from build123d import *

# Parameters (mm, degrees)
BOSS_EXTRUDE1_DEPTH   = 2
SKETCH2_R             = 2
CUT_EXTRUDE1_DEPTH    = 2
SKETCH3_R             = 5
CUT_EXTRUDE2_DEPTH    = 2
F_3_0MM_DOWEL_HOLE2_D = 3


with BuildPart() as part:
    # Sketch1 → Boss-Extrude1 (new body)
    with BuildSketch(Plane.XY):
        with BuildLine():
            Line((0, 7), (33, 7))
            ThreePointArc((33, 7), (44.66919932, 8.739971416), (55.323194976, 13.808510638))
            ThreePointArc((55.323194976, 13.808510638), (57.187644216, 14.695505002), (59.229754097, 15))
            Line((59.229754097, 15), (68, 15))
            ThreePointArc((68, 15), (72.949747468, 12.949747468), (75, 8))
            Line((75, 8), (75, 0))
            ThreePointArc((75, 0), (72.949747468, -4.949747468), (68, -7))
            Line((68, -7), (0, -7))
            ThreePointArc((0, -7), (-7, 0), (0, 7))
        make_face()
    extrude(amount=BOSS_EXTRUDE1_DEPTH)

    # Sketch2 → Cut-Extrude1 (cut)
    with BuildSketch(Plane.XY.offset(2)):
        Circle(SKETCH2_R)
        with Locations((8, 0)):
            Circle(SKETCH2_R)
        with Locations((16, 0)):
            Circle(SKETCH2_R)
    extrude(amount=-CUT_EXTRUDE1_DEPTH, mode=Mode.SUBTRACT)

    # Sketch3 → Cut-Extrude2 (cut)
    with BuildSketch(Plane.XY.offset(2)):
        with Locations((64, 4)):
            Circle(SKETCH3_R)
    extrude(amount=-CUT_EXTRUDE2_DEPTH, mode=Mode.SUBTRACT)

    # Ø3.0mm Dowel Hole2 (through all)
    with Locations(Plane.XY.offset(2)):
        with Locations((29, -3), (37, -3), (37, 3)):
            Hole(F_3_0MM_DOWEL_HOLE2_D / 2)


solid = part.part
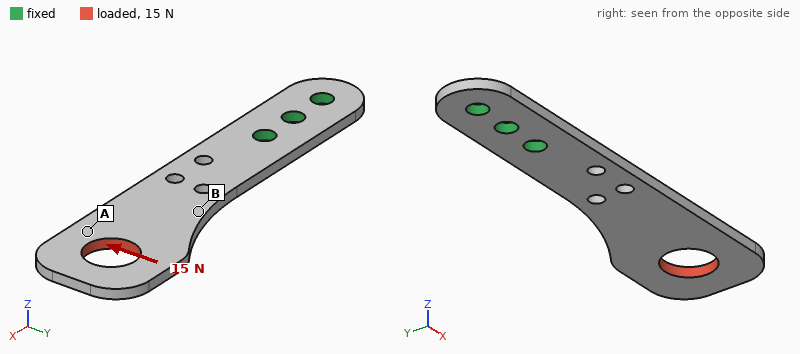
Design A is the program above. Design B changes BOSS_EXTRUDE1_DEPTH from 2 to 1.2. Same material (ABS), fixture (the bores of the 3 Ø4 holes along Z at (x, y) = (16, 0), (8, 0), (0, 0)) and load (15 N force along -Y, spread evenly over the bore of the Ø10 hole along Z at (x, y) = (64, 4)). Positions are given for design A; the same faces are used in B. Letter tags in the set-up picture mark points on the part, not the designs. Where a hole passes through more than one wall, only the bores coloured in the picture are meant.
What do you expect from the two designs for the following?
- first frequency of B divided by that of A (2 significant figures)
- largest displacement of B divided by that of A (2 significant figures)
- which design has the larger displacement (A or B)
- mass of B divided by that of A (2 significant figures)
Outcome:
0.61
1.7
B
0.60
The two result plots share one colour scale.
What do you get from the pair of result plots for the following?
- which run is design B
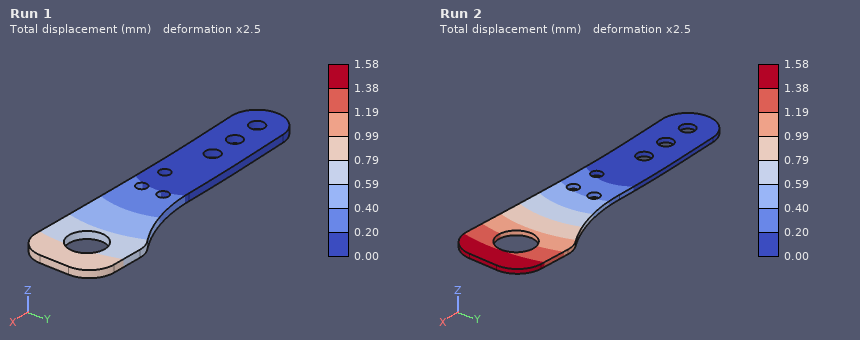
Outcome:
Run 2
